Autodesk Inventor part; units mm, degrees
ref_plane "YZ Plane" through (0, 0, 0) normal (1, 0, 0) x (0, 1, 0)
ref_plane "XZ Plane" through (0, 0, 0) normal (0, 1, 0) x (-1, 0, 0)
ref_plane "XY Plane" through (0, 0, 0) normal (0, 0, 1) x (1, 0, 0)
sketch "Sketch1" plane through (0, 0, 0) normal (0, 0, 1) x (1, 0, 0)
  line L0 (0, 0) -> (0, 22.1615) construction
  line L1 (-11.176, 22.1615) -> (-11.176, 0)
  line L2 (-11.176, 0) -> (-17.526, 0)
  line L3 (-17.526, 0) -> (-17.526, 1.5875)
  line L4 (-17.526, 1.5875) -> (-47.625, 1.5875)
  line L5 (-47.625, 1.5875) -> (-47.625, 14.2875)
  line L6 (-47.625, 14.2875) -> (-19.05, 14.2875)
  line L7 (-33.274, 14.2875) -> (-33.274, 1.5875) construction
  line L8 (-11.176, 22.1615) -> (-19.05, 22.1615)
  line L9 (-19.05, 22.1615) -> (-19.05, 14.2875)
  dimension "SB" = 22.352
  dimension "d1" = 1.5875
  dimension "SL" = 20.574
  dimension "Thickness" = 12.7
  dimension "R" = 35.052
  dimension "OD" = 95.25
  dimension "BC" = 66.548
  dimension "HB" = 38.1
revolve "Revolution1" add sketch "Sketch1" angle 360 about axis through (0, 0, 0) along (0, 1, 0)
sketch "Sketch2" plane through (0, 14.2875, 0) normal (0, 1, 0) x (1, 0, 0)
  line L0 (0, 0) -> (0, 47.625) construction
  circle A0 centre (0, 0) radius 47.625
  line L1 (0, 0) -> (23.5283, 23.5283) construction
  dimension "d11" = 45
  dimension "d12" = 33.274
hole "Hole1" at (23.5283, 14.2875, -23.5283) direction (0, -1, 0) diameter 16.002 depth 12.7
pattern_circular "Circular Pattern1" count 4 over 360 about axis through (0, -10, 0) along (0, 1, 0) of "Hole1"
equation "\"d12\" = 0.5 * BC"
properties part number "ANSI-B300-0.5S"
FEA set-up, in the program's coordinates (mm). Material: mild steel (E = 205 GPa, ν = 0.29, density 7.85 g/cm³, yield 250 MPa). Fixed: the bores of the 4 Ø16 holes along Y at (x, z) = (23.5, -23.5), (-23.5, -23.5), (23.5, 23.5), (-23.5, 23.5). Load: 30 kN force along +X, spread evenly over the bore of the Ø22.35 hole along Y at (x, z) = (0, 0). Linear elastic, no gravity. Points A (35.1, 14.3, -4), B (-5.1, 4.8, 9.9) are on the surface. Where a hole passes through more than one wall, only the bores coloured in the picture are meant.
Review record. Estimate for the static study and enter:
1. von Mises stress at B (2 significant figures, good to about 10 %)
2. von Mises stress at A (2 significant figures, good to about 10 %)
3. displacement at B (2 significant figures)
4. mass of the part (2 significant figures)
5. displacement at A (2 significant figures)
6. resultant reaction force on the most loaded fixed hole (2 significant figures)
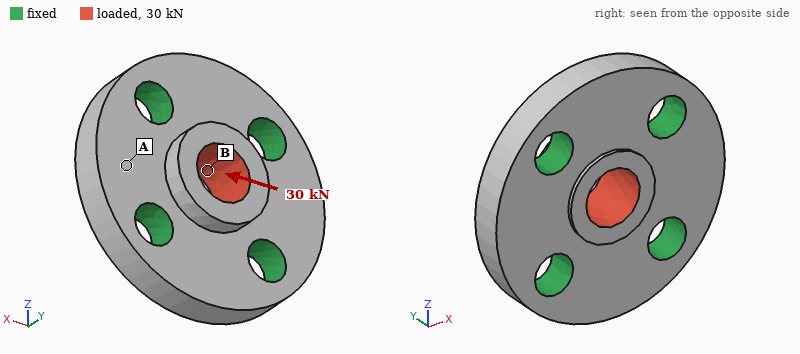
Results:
33 MPa
7.8 MPa
2.3 µm
640 g
1.3 µm
8.0 kN
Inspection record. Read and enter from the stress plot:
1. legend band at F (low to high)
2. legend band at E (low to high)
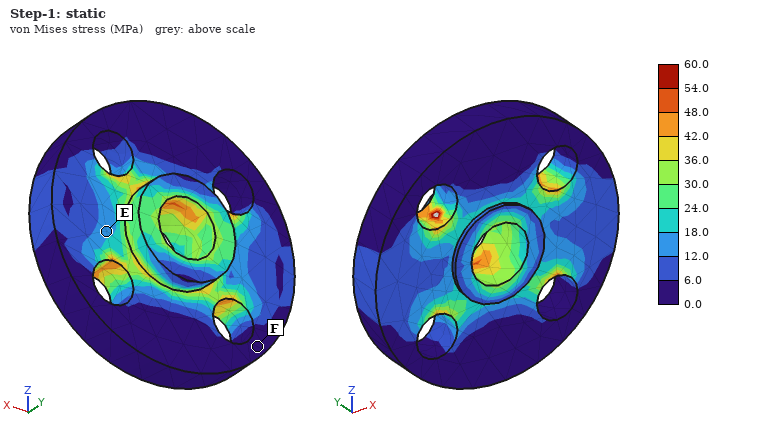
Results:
0.0 to 6.0 MPa
12.0 to 18.0 MPa
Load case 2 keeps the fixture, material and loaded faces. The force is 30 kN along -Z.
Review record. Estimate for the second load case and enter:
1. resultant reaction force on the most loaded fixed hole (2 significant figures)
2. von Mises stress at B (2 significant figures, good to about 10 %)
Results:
8.0 kN
24 MPa
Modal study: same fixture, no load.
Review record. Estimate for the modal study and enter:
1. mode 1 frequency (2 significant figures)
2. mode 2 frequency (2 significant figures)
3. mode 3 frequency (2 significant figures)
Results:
21 kHz
21 kHz
21 kHz
